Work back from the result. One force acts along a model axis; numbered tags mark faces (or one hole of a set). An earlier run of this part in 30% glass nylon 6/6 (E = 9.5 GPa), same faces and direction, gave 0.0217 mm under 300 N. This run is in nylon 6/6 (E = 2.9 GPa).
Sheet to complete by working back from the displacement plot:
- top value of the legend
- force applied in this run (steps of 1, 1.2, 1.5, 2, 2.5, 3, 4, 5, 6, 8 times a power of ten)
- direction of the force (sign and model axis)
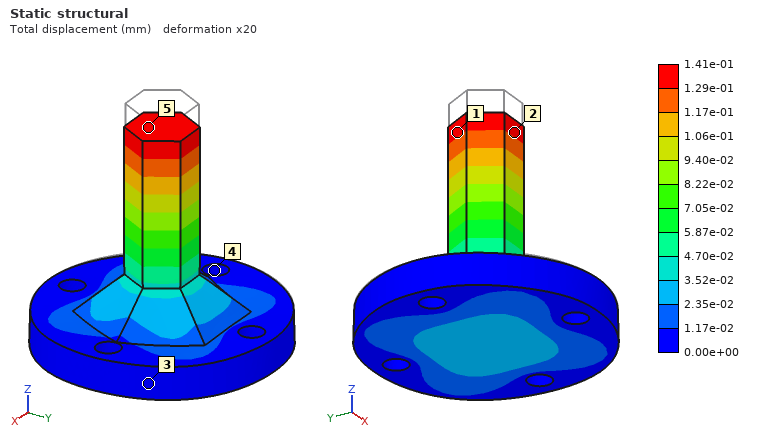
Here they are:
1.41e-01 mm
600 N
-Z
